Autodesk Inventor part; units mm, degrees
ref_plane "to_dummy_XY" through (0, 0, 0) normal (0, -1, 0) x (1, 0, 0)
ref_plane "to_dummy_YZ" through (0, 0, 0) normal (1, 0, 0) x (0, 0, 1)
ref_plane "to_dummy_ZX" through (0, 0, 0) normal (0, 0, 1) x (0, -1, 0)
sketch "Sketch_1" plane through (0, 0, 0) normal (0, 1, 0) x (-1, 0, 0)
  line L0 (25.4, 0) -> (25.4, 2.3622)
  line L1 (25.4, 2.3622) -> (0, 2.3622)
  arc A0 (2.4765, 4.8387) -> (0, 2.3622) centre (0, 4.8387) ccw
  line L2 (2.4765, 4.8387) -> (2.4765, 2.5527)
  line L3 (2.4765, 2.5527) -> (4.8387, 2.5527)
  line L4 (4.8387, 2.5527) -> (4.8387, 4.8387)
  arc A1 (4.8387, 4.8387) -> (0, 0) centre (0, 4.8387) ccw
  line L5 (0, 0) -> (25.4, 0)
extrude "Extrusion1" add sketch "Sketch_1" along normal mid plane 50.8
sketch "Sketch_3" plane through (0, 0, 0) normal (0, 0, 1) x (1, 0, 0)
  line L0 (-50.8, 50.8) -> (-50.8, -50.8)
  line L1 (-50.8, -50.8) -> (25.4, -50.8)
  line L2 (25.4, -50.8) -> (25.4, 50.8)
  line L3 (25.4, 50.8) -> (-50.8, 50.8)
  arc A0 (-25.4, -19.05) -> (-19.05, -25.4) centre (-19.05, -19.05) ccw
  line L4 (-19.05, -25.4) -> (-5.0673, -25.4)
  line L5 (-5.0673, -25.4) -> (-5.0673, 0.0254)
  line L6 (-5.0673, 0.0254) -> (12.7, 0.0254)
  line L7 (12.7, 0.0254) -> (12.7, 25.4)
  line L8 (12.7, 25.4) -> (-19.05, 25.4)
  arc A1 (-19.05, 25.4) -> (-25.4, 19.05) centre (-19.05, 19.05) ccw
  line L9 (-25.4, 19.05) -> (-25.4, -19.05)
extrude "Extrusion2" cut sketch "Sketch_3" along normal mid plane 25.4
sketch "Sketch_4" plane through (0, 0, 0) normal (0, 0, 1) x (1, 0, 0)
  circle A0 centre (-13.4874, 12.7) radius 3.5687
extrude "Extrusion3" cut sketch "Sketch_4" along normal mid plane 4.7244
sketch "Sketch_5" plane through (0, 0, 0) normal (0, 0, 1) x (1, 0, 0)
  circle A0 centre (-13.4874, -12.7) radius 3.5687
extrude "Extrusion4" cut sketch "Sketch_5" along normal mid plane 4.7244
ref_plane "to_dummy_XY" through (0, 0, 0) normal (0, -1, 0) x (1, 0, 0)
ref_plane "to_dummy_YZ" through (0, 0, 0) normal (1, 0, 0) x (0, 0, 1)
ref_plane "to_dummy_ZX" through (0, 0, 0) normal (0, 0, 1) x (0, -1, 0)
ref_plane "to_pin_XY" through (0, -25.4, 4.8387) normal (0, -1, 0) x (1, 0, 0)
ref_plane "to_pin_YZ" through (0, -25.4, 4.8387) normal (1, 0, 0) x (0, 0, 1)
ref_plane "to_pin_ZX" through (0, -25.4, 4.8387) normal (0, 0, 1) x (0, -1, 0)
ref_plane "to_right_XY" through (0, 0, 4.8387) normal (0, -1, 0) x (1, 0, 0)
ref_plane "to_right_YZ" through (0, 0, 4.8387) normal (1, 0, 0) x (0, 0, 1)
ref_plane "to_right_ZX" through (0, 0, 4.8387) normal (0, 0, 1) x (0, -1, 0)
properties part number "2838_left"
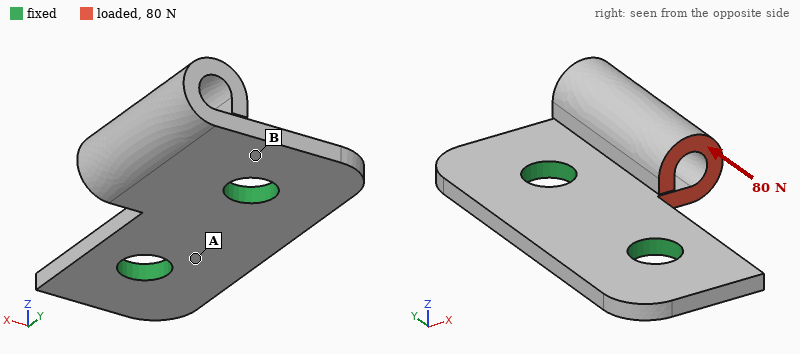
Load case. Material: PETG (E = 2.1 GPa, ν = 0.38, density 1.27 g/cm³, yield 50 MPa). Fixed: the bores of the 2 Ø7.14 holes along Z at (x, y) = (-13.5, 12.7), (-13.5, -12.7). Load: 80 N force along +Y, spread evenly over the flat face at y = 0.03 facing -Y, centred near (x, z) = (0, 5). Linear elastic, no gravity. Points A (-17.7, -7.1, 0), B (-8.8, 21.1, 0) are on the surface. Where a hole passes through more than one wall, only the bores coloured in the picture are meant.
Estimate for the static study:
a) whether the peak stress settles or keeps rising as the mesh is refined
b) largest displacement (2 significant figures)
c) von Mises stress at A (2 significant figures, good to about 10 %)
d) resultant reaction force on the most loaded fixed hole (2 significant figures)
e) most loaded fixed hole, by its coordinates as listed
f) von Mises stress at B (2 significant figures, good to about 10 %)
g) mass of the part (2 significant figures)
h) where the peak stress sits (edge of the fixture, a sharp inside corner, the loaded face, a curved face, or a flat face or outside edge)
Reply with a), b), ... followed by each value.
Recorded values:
a) keeps rising
b) 0.53 mm
c) 1.8 MPa
d) 65 N
e) (-13.5, 12.7)
f) 5.7 MPa
g) 4.7 g
h) a sharp inside corner
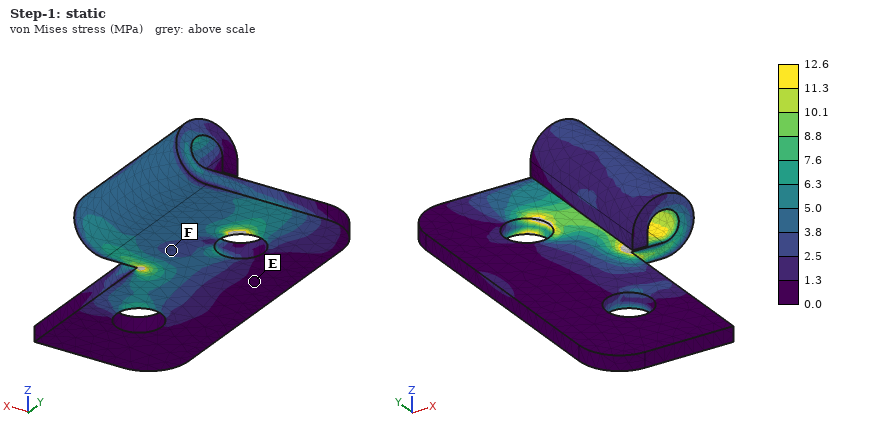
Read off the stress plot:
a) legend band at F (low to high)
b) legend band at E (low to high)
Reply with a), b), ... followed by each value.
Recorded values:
a) 2.5 to 3.8 MPa
b) 0.0 to 1.3 MPa
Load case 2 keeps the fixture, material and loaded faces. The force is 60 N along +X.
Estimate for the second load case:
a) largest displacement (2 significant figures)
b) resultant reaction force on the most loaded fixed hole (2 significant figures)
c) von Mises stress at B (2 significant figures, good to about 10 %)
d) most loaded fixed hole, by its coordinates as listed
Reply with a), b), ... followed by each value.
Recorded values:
a) 0.72 mm
b) 36 N
c) 5.1 MPa
d) (-13.5, 12.7)
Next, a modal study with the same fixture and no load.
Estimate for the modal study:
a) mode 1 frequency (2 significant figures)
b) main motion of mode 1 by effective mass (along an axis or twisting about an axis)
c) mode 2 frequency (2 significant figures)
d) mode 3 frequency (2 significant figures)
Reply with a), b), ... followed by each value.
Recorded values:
a) 1100 Hz
b) along Z
c) 1400 Hz
d) 2000 Hz
